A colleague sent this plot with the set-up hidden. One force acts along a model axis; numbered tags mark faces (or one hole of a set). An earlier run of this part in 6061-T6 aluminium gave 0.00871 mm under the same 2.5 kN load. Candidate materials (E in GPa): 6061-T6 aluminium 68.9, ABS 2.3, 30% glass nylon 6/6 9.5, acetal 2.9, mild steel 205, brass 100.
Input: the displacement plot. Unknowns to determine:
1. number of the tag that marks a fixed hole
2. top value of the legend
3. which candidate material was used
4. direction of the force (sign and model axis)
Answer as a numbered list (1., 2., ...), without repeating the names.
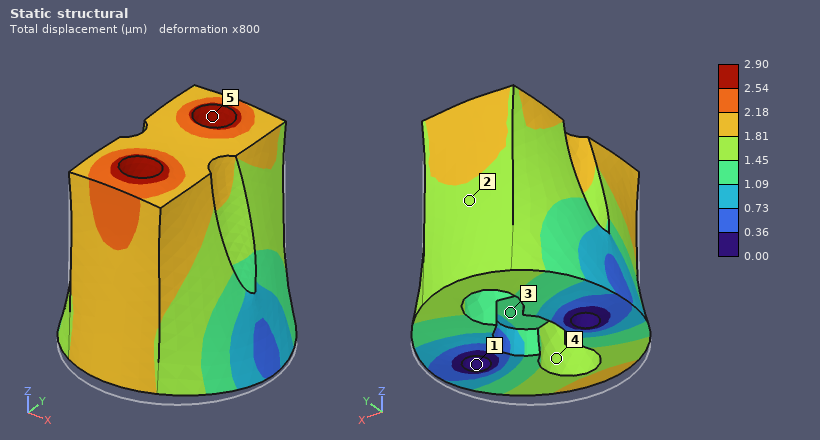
1. 1
2. 2.90 µm
3. mild steel
4. +Z
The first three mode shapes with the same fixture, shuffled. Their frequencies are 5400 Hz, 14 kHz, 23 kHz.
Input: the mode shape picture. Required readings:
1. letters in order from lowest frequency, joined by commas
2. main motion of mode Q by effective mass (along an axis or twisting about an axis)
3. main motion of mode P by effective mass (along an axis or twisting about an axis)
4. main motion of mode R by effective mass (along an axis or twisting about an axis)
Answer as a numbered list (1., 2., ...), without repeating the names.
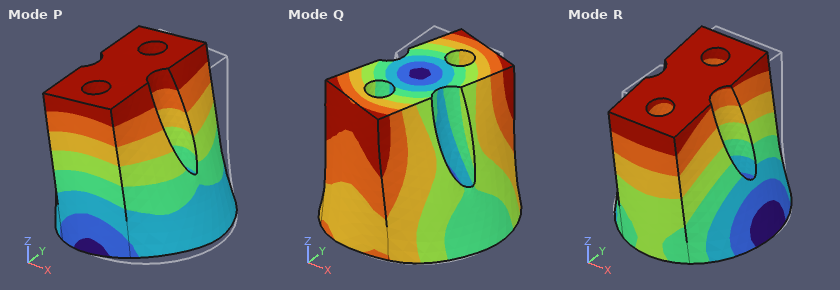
1. R, P, Q
2. twisting about Z
3. along X
4. along Y
